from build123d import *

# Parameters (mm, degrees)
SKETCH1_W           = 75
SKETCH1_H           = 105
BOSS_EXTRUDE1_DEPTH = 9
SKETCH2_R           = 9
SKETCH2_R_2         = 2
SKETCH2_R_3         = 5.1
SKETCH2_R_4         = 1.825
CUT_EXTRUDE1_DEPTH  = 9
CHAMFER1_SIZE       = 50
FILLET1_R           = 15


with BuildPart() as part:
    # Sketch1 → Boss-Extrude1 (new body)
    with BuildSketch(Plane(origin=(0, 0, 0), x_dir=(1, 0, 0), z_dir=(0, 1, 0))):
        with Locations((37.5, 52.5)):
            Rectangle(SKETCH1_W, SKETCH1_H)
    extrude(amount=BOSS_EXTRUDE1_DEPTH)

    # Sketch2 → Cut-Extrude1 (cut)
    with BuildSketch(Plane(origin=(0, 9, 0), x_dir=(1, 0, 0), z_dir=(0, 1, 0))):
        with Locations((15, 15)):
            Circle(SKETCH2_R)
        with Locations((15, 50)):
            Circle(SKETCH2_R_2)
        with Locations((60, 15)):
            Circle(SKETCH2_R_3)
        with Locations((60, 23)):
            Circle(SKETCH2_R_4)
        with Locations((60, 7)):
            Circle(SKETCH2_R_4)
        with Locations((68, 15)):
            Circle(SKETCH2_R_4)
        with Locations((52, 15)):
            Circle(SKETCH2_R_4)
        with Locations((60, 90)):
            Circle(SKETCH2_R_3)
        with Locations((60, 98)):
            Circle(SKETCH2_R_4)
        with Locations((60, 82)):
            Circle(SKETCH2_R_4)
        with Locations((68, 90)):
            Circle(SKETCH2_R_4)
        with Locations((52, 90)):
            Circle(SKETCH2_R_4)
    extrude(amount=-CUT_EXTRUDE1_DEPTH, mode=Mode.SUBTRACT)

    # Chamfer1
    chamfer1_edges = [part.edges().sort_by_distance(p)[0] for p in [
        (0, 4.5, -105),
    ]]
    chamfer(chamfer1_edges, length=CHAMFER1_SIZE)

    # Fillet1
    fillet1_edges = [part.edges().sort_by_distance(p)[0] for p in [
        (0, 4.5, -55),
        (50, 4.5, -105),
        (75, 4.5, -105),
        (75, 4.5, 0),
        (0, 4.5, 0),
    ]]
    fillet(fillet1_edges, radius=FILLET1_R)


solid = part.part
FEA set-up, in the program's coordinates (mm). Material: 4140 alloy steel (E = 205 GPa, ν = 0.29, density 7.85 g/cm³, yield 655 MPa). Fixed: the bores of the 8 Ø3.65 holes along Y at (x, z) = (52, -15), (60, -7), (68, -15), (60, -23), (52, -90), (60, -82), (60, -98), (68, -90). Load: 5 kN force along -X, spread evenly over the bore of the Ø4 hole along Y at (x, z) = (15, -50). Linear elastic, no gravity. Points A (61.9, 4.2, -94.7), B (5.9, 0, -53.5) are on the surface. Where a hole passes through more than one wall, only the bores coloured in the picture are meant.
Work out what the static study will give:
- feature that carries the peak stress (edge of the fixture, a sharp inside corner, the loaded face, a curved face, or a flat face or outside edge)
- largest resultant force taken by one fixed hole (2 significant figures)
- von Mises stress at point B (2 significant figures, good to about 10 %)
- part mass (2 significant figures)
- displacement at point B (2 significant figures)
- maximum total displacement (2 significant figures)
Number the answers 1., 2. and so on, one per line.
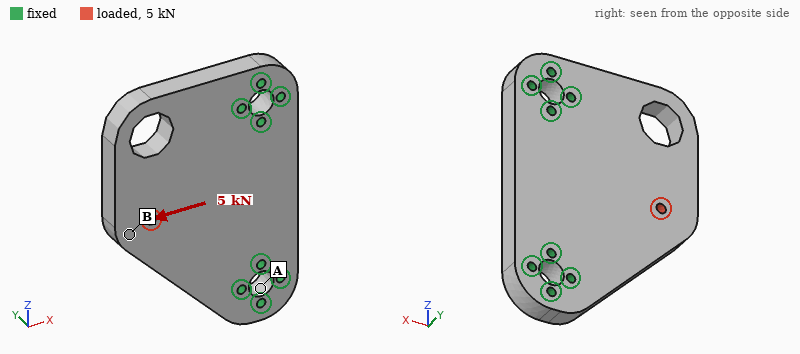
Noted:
1. the loaded face
2. 1.6 kN
3. 16 MPa
4. 420 g
5. 3.7 µm
6. 4.6 µm
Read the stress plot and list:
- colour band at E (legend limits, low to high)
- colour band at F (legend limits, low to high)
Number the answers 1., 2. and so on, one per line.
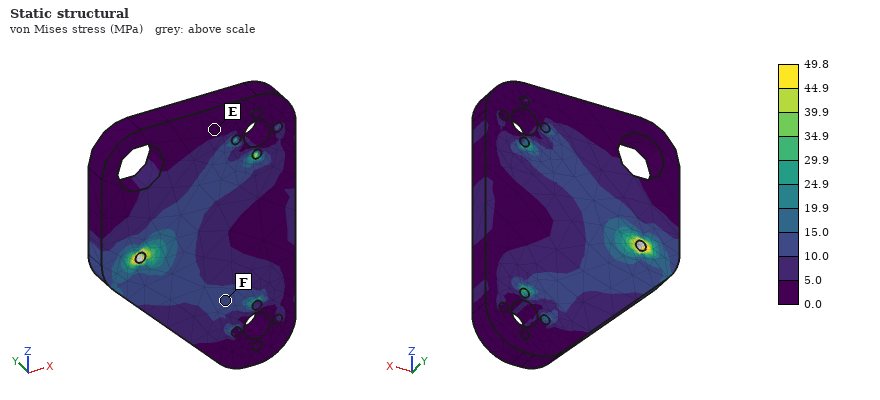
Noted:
1. 0.0 to 5.0 MPa
2. 10.0 to 15.0 MPa
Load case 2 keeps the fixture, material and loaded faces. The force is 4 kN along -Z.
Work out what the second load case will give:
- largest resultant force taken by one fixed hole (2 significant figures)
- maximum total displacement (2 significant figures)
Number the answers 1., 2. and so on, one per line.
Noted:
1. 1.6 kN
2. 5.1 µm
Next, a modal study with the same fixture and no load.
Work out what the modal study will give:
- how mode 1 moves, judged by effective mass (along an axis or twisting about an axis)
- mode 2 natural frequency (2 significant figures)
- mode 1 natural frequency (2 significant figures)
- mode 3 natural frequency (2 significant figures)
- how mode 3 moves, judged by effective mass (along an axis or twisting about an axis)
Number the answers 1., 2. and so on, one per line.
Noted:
1. along Y
2. 5800 Hz
3. 2600 Hz
4. 10 kHz
5. along Y
